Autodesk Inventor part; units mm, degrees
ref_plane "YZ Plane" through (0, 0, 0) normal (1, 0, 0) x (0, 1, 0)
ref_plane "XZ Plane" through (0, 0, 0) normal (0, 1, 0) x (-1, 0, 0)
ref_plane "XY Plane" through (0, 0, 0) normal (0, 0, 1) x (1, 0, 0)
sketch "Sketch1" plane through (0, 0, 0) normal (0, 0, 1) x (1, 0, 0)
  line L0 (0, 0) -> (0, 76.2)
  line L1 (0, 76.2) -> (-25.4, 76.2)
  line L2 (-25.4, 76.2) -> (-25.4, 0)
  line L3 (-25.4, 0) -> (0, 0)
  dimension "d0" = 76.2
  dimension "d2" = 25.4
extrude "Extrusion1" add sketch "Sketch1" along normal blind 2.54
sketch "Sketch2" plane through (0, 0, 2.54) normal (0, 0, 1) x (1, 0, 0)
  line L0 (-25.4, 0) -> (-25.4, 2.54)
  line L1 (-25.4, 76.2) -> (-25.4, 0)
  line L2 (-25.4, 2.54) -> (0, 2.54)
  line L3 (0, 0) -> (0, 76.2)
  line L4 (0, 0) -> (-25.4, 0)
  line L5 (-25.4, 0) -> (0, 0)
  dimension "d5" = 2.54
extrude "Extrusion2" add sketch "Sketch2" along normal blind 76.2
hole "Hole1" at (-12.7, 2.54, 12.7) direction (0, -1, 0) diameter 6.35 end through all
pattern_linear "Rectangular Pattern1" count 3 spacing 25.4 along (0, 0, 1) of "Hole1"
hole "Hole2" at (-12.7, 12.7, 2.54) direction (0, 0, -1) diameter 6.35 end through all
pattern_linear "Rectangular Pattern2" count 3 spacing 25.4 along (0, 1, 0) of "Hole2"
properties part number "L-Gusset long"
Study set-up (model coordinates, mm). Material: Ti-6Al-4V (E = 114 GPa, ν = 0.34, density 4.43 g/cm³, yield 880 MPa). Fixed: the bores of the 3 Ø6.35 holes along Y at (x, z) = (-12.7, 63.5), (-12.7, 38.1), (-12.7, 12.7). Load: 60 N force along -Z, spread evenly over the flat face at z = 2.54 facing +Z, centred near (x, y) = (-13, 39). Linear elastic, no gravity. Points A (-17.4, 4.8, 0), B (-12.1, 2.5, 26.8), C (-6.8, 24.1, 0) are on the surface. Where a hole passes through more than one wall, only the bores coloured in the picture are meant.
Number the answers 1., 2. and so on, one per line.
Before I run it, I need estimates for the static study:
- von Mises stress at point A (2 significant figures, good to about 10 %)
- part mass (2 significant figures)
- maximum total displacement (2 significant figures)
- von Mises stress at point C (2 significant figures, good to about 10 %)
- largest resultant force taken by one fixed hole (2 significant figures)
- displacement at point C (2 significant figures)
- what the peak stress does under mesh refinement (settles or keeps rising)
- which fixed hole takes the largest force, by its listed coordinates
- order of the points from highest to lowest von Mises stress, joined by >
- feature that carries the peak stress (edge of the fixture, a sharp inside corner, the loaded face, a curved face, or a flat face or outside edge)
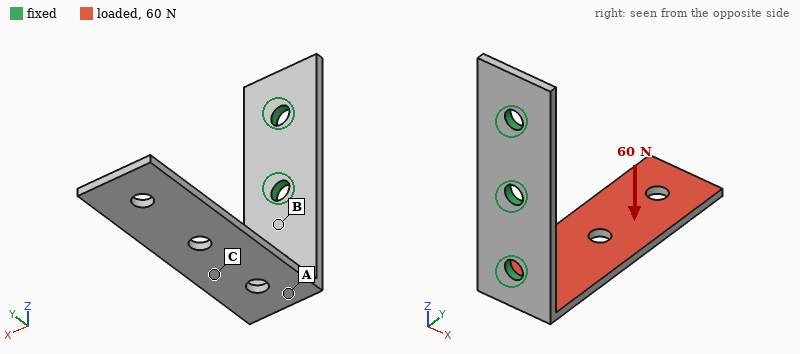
1. 68 MPa
2. 41 g
3. 1.2 mm
4. 39 MPa
5. 60 N
6. 0.25 mm
7. keeps rising
8. (-12.7, 12.7)
9. A > C > B
10. edge of the fixture
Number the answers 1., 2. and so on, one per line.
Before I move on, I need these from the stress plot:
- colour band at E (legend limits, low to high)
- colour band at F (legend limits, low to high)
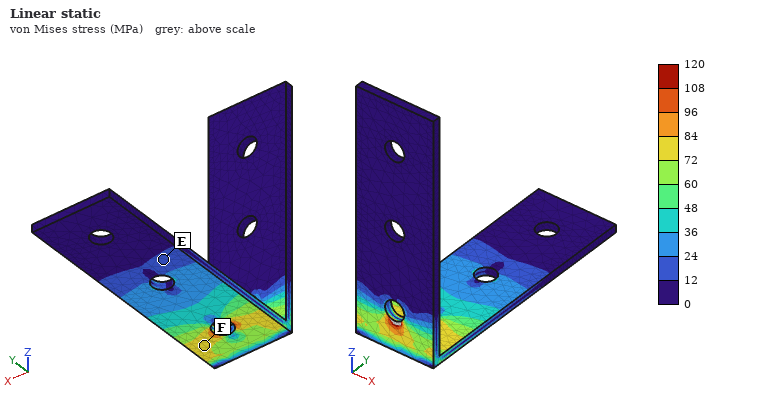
1. 12 to 24 MPa
2. 72 to 84 MPa
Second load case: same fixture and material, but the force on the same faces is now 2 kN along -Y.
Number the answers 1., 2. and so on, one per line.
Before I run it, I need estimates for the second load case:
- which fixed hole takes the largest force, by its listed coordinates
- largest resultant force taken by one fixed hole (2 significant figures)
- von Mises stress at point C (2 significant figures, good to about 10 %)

1. (-12.7, 12.7)
2. 2.1 kN
3. 41 MPa
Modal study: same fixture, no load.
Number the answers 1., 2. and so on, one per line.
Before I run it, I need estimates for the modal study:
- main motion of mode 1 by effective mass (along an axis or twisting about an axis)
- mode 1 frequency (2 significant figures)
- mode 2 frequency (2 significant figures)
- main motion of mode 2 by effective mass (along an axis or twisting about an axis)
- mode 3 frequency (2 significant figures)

1. along Z
2. 310 Hz
3. 730 Hz
4. along X
5. 1900 Hz
